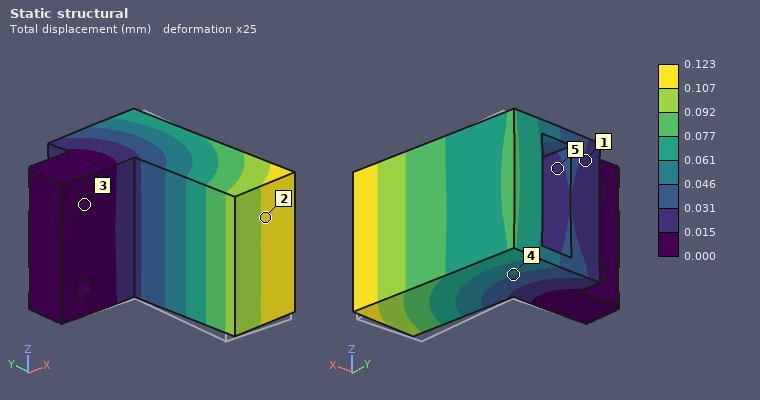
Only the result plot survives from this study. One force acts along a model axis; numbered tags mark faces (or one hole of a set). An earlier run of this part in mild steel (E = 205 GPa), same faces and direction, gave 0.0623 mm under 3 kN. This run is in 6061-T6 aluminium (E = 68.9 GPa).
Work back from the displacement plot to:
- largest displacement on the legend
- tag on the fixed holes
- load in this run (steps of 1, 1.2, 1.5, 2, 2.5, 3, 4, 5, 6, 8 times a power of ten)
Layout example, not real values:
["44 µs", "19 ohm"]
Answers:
["0.123 mm", "3", "2 kN"]
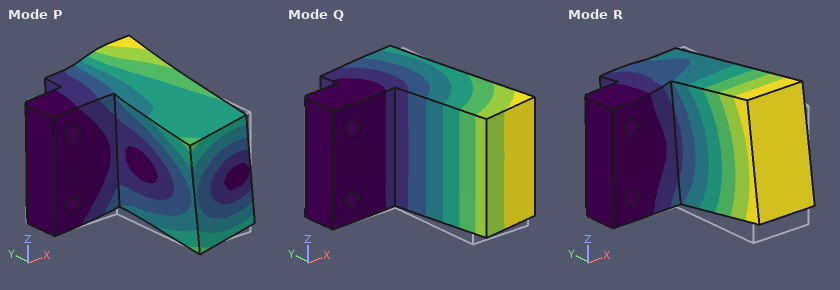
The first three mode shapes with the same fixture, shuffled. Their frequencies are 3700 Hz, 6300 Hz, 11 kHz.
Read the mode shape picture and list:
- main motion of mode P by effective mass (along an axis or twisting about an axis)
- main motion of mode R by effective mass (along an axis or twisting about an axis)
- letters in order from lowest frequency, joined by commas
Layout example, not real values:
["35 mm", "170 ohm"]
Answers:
["along Z", "along Z", "Q, R, P"]
